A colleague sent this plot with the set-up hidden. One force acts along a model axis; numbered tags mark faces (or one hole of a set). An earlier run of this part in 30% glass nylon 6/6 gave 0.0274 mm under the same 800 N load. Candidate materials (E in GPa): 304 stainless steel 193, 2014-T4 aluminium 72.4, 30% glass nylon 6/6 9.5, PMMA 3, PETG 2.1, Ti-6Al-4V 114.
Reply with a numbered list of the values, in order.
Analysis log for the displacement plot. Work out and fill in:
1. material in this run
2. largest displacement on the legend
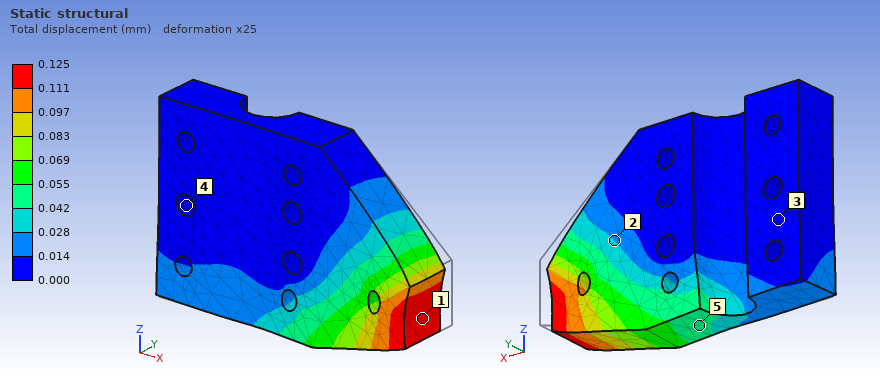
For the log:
1. PETG
2. 0.125 mm
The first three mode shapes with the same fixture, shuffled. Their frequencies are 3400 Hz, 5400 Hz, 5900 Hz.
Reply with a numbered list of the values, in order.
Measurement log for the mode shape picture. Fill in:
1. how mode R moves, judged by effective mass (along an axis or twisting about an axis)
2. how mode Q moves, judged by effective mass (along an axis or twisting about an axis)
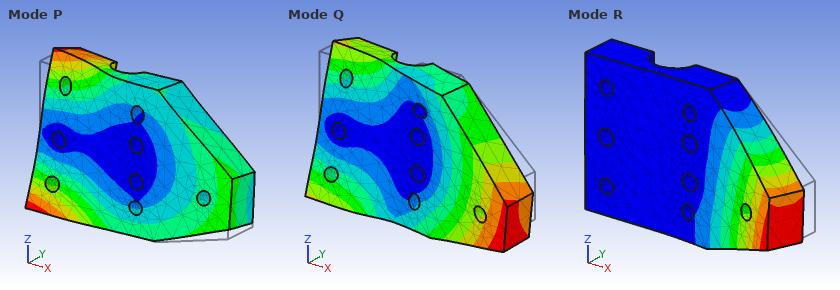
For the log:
1. along Y
2. along Z
